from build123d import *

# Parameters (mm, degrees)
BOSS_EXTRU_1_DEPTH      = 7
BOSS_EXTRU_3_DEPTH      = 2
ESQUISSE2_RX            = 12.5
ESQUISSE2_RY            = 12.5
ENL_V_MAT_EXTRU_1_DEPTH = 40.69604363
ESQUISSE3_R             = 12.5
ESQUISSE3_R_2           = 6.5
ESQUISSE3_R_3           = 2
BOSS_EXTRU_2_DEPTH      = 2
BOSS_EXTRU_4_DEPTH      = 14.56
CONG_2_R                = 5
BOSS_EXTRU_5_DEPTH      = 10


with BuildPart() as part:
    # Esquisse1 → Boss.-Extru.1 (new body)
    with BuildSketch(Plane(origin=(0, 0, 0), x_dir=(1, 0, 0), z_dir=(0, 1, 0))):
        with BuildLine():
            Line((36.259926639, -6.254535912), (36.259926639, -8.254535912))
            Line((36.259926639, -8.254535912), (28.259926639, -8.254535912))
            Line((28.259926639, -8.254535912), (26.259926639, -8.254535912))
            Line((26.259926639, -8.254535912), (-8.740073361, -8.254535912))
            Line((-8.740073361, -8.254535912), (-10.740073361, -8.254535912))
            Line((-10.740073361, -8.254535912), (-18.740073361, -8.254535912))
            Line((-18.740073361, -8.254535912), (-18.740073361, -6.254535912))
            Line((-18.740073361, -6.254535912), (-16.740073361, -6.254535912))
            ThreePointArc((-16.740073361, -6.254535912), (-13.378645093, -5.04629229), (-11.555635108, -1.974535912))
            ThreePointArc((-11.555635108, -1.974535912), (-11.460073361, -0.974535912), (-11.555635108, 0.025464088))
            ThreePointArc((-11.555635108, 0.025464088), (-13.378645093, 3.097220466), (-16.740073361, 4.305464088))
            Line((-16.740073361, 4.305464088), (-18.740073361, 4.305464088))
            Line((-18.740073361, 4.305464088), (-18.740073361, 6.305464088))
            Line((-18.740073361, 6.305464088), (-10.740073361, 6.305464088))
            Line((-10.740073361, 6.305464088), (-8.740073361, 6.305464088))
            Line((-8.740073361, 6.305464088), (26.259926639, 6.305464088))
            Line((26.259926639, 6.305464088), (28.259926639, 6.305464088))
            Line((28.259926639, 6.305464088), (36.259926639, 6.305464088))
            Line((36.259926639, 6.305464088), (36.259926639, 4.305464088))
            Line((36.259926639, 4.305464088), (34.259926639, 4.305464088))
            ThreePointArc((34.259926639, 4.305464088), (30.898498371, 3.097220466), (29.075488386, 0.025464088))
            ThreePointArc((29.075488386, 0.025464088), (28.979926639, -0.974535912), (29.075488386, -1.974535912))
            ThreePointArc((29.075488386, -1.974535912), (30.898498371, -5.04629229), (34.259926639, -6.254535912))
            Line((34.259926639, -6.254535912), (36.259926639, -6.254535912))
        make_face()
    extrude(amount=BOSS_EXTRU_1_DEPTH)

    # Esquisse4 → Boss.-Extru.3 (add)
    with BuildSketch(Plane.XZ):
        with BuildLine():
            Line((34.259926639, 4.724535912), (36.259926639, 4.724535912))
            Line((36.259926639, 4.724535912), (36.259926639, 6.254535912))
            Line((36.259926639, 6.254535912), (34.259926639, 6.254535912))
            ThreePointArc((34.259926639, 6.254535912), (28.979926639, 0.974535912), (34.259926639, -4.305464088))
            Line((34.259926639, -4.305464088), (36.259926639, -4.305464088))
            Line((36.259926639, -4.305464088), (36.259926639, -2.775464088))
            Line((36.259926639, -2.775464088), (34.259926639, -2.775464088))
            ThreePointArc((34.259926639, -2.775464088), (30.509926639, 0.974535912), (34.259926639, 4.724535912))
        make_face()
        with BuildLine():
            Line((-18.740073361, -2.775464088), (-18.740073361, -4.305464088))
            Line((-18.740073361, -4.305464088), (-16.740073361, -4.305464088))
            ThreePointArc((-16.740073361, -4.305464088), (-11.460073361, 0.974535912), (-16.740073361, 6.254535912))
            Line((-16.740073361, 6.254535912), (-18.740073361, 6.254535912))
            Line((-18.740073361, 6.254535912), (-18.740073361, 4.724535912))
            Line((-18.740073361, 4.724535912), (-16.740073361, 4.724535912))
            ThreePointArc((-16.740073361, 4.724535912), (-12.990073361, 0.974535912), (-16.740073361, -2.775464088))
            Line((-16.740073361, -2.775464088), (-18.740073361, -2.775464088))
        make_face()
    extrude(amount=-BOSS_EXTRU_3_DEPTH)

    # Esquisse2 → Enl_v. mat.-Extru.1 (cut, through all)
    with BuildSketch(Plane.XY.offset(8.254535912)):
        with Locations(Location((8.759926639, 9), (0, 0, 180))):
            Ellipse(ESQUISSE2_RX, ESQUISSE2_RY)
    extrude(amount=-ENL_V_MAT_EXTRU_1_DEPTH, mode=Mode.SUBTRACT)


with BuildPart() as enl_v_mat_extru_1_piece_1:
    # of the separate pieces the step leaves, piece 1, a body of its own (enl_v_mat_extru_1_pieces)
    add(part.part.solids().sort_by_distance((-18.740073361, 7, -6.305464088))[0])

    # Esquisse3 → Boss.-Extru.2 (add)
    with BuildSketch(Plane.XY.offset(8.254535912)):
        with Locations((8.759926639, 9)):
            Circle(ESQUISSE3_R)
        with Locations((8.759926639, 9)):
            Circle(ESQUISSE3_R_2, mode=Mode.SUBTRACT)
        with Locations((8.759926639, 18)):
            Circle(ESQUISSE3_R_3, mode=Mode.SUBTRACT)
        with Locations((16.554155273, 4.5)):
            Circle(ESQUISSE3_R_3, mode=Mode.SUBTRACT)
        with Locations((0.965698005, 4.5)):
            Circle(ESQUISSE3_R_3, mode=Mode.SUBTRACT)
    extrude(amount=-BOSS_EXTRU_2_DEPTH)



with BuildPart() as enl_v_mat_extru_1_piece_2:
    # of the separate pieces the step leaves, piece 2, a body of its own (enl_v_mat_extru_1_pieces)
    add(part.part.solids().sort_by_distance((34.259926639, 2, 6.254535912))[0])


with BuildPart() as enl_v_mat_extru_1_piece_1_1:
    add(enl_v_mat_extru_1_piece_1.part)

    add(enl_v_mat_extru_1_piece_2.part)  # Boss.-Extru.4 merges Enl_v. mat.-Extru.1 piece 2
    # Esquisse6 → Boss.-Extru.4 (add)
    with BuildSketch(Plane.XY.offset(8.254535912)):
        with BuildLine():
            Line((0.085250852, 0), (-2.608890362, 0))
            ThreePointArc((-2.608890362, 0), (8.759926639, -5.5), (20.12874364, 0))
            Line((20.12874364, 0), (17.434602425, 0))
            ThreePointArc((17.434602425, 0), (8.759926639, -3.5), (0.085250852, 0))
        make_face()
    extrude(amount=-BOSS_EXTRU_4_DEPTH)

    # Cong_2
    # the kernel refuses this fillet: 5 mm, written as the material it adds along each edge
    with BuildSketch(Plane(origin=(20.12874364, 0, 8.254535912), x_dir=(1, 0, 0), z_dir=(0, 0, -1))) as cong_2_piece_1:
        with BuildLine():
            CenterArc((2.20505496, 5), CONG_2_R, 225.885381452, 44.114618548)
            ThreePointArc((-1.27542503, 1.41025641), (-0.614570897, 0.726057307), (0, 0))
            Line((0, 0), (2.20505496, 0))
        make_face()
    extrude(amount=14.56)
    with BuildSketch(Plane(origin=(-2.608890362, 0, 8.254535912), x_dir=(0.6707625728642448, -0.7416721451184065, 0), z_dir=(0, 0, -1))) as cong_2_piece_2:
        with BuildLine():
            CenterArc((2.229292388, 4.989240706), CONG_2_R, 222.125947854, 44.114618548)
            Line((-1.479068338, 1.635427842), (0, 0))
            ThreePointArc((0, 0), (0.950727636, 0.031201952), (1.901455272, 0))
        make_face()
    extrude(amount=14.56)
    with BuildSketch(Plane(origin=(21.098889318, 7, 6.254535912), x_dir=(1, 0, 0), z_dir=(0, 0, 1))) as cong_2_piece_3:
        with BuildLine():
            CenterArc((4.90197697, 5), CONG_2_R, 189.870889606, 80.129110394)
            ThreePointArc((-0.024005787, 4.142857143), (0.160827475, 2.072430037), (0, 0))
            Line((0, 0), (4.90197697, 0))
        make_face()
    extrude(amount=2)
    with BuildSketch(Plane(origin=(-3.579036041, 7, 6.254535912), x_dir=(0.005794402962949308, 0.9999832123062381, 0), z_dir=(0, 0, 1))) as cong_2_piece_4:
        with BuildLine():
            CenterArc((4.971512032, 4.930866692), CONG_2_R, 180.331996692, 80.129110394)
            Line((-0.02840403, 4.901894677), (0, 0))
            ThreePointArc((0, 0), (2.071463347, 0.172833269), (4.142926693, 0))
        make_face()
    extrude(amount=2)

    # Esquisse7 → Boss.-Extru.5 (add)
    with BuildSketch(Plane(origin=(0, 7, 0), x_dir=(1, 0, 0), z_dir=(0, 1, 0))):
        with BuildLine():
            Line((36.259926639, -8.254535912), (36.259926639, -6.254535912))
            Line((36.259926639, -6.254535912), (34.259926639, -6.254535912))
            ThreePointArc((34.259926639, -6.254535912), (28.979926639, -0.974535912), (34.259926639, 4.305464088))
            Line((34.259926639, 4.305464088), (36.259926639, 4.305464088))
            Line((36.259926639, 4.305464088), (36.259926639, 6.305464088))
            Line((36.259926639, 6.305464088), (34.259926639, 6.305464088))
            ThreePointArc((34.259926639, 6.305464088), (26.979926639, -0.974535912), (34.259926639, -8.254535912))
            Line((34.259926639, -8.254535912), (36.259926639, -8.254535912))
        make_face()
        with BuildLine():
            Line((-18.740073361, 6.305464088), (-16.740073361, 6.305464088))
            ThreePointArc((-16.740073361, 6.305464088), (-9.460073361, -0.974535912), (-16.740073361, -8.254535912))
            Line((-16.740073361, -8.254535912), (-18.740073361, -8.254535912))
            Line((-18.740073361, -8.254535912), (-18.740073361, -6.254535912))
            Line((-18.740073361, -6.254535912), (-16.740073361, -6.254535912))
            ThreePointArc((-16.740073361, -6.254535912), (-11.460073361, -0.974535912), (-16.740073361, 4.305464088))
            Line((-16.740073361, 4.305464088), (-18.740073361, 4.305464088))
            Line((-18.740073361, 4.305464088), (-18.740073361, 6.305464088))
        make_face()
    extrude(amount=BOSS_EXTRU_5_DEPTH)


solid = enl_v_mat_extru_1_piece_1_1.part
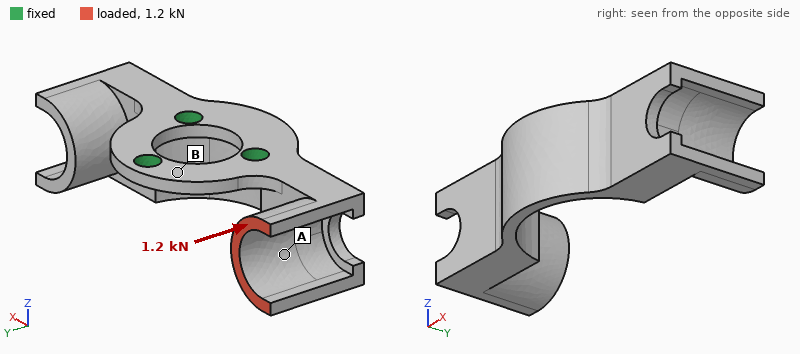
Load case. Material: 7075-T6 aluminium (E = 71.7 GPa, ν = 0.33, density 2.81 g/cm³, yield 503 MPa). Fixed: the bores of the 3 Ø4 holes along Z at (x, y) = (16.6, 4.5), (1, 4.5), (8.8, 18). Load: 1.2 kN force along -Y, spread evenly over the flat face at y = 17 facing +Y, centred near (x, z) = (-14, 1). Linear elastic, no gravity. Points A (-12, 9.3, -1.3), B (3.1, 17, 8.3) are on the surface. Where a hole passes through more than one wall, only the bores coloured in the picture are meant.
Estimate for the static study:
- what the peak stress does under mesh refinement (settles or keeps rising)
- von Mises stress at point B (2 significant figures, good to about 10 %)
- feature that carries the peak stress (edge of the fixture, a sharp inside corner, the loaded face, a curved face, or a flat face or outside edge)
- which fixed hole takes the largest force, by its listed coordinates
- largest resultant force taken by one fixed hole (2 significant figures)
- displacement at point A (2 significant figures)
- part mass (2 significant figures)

keeps rising
98 MPa
edge of the fixture
(1, 4.5)
1.1 kN
0.27 mm
14 g
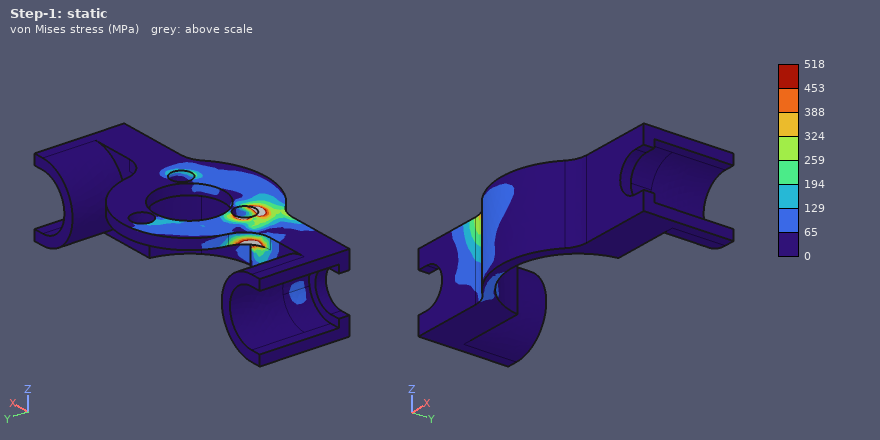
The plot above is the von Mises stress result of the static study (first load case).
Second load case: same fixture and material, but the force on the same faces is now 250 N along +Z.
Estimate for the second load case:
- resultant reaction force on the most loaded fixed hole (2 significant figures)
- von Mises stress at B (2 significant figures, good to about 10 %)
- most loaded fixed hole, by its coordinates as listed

390 N
21 MPa
(1, 4.5)
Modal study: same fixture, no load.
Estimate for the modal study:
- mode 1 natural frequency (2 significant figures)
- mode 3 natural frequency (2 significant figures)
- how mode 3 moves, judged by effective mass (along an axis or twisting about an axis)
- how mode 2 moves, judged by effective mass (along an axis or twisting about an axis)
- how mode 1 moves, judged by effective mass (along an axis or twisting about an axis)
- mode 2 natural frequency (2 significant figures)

3800 Hz
5100 Hz
along Z
along Y
along X
4600 Hz
